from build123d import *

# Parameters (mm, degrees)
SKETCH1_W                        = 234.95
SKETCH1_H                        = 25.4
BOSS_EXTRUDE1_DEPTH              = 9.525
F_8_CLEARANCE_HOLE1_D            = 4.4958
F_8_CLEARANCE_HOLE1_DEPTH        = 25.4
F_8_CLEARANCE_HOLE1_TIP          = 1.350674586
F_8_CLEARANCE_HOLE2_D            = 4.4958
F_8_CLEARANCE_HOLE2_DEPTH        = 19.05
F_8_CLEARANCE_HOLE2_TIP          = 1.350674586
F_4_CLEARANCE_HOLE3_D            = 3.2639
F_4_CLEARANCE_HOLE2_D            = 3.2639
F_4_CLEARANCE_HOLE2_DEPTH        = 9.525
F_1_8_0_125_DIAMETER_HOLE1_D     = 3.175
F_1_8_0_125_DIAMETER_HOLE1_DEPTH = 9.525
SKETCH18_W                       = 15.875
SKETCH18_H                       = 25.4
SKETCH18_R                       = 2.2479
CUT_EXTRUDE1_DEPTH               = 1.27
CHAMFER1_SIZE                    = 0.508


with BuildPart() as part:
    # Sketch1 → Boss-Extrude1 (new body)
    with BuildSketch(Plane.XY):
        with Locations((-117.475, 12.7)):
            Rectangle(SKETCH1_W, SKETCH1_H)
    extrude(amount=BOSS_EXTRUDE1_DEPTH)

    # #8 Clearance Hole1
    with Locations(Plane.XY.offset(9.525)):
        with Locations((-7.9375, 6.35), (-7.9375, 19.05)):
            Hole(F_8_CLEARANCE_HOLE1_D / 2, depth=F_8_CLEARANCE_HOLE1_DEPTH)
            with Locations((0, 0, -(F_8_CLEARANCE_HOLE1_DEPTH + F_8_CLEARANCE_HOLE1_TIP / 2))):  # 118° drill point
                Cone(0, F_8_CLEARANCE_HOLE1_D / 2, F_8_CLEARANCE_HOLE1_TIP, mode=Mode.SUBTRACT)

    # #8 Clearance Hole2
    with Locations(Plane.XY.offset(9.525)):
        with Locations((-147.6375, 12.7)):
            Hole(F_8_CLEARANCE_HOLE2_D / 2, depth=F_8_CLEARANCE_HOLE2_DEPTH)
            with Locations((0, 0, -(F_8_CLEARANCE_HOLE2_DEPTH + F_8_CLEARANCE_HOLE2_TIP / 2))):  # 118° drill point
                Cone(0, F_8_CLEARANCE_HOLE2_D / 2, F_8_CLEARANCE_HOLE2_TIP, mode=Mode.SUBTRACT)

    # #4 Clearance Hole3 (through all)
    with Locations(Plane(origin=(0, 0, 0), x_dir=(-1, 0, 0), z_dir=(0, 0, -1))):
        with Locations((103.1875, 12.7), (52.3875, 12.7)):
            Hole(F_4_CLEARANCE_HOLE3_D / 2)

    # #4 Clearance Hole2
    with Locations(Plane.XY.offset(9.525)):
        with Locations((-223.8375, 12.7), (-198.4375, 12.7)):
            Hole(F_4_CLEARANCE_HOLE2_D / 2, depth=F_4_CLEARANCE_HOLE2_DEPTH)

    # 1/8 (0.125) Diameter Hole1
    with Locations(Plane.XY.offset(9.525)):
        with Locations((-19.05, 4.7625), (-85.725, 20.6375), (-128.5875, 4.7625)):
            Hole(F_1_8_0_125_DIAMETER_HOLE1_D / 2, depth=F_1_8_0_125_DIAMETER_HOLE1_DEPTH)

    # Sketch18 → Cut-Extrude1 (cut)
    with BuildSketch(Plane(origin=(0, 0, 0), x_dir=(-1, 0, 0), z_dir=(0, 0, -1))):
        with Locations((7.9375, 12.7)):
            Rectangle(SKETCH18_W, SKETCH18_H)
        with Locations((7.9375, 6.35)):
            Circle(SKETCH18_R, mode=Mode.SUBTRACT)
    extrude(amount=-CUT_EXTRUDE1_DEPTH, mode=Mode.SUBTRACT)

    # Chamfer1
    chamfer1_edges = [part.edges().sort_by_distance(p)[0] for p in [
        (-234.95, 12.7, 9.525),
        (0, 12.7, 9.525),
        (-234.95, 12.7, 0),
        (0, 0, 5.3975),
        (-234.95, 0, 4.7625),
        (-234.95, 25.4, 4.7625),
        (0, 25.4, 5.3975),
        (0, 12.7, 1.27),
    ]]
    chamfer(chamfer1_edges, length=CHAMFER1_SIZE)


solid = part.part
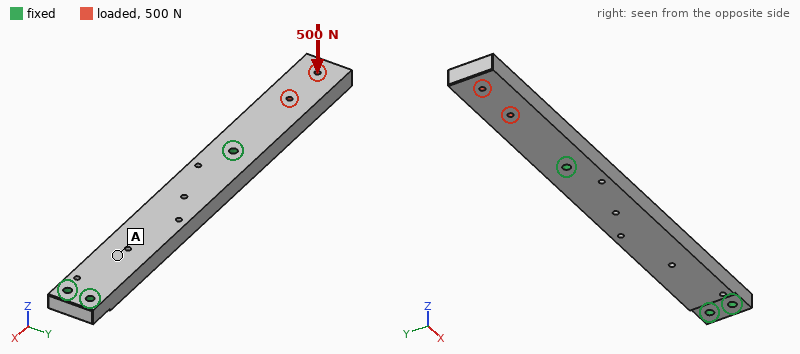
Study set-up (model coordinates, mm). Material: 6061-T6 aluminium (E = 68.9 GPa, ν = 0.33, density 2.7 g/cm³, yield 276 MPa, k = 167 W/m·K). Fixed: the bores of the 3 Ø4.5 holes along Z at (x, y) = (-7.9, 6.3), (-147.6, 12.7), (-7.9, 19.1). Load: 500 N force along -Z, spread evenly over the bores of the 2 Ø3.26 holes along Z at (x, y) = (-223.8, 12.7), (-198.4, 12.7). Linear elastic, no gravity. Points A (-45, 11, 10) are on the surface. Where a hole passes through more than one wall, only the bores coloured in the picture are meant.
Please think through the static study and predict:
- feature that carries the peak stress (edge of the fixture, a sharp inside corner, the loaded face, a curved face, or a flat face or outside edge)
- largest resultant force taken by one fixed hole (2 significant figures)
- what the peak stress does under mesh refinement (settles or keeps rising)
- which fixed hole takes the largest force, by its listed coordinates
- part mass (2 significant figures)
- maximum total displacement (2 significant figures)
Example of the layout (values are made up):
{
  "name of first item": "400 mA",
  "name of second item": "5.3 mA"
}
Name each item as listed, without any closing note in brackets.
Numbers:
{
  "feature that carries the peak stress": "edge of the fixture",
  "largest resultant force taken by one fixed hole": "520 N",
  "what the peak stress does under mesh refinement": "keeps rising",
  "which fixed hole takes the largest force, by its listed coordinates": "(-147.6, 12.7)",
  "part mass": "150 g",
  "maximum total displacement": "0.58 mm"
}
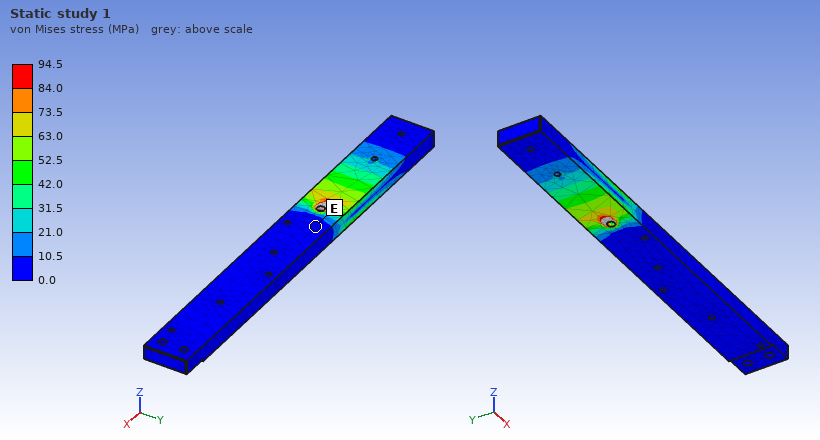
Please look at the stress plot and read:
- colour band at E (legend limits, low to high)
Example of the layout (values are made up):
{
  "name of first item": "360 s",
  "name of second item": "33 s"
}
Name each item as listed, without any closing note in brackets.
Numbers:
{
  "colour band at E": "0.0 to 10.5 MPa"
}
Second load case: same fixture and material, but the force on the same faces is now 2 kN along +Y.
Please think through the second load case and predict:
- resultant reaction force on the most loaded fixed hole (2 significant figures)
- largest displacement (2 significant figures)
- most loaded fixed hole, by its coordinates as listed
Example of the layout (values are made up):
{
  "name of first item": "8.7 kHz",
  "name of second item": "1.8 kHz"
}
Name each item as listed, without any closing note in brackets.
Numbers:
{
  "resultant reaction force on the most loaded fixed hole": "2.7 kN",
  "largest displacement": "0.61 mm",
  "most loaded fixed hole, by its coordinates as listed": "(-147.6, 12.7)"
}
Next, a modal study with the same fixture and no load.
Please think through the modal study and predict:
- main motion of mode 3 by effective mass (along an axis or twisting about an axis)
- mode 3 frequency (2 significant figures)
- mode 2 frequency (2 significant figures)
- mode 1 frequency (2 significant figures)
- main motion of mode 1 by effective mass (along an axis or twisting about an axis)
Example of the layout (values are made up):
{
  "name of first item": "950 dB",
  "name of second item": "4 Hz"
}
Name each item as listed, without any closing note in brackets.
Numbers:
{
  "main motion of mode 3 by effective mass": "along Z",
  "mode 3 frequency": "2300 Hz",
  "mode 2 frequency": "1800 Hz",
  "mode 1 frequency": "980 Hz",
  "main motion of mode 1 by effective mass": "along Z"
}
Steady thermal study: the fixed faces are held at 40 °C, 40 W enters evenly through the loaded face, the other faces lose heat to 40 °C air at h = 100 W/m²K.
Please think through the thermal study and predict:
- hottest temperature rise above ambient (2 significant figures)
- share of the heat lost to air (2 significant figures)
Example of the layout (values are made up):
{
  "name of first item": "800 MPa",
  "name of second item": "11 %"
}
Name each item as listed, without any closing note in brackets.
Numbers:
{
  "hottest temperature rise above ambient": "44 K",
  "share of the heat lost to air": "43 %"
}
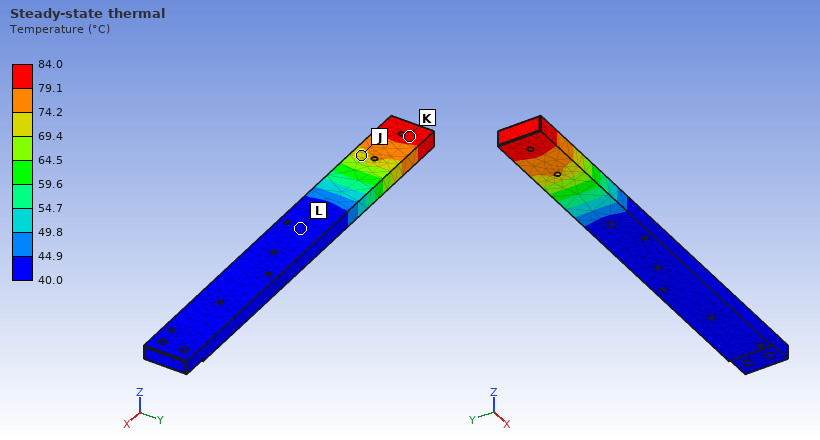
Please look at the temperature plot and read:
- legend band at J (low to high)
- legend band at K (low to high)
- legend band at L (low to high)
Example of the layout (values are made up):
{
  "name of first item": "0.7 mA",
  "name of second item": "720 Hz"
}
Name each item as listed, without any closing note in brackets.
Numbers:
{
  "legend band at J": "69.4 to 74.2 °C",
  "legend band at K": "79.1 to 84.0 °C",
  "legend band at L": "40.0 to 44.9 °C"
}
